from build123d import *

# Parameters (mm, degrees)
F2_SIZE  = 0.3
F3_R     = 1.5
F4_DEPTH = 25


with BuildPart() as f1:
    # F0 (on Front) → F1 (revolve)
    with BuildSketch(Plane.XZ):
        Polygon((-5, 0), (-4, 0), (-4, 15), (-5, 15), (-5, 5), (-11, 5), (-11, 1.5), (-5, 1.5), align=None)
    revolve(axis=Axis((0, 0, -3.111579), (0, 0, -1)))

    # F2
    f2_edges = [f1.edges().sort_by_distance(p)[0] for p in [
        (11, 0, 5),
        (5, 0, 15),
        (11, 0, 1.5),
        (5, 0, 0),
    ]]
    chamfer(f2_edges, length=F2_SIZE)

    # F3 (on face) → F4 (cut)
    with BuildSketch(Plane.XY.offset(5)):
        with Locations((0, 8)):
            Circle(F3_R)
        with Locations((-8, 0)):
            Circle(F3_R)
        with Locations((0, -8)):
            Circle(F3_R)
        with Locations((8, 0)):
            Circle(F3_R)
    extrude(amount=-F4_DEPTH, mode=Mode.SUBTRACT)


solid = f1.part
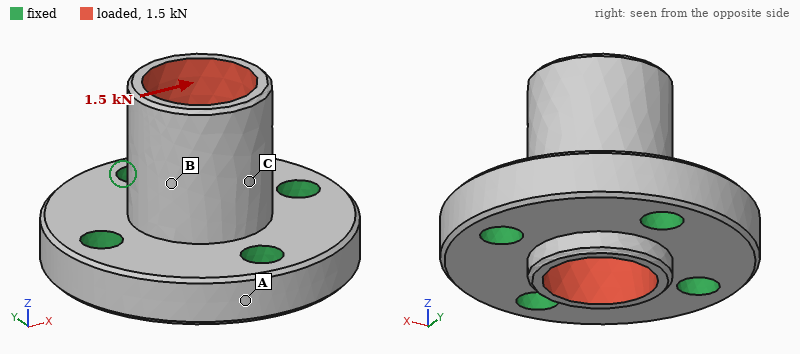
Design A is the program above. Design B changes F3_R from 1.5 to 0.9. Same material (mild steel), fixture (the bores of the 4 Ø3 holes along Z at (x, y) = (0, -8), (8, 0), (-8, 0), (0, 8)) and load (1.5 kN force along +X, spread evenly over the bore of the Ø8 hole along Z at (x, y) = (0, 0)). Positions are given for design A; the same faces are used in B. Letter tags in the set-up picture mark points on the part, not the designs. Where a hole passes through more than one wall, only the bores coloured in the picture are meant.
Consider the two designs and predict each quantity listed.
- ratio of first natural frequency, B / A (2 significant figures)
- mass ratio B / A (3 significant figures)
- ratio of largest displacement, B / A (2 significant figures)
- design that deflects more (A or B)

0.95
1.05
1.1
B
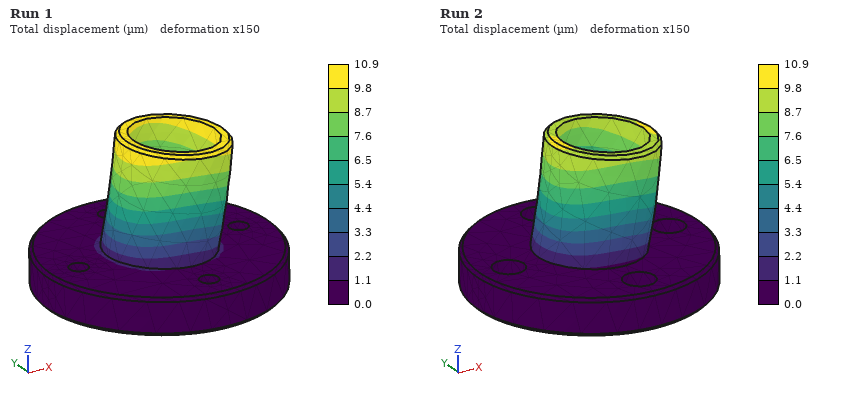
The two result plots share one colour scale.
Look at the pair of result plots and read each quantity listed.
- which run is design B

Run 1
